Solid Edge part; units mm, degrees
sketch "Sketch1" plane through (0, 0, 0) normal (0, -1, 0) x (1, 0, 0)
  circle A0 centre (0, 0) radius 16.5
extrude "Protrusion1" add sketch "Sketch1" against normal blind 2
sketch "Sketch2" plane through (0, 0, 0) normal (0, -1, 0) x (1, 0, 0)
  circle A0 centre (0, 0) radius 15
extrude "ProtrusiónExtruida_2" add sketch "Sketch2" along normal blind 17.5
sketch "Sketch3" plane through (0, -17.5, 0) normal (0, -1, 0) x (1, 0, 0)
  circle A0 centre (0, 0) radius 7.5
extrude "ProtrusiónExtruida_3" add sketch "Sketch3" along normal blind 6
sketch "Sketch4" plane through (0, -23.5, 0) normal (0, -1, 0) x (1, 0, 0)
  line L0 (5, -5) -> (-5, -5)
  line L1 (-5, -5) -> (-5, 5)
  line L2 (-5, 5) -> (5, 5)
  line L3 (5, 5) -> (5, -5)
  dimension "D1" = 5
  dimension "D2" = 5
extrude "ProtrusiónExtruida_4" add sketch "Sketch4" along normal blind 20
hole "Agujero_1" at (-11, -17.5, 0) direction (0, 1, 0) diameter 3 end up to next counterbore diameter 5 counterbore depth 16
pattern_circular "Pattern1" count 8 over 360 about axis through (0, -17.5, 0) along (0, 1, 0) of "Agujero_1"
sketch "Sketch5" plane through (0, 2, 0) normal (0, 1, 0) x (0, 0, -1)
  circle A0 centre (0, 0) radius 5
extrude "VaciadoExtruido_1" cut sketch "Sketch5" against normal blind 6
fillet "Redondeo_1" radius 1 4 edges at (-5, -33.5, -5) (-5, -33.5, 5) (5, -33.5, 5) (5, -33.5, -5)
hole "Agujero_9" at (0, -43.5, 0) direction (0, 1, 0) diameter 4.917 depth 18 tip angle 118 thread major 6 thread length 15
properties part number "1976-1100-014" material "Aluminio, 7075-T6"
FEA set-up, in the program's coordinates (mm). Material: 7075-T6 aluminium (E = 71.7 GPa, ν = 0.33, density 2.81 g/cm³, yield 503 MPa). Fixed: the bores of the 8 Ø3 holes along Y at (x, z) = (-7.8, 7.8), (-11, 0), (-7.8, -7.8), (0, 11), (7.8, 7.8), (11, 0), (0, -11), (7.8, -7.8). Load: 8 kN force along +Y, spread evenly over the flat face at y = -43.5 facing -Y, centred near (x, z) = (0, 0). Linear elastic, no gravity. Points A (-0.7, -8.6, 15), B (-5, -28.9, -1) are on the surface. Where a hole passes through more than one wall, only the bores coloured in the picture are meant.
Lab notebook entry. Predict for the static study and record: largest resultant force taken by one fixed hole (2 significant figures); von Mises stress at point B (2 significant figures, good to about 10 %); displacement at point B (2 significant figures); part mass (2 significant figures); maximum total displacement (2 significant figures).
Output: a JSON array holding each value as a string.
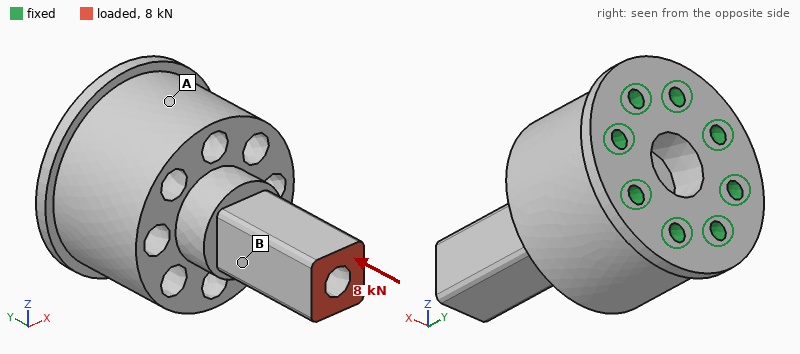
["1.1 kN", "98 MPa", "20 µm", "38 g", "40 µm"]
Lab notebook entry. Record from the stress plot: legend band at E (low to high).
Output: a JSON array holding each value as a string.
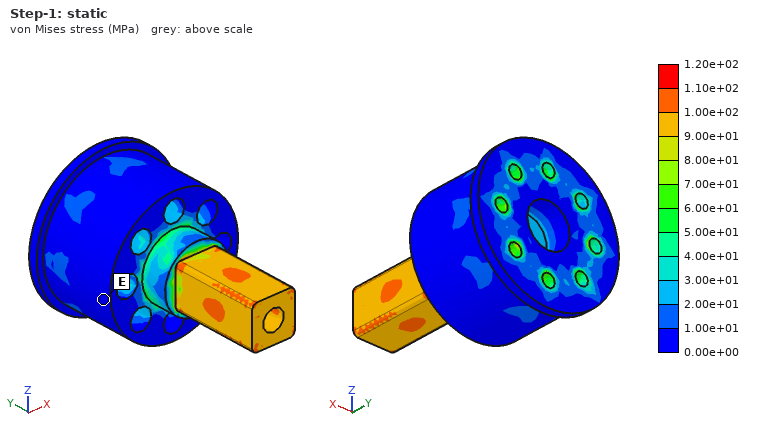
["0.00e+00 to 1.00e+01 MPa"]
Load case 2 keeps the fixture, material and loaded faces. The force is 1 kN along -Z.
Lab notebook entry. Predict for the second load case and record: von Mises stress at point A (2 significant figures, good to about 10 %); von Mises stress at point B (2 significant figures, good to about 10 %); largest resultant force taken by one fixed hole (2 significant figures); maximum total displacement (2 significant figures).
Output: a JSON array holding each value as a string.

["12 MPa", "44 MPa", "940 N", "0.12 mm"]
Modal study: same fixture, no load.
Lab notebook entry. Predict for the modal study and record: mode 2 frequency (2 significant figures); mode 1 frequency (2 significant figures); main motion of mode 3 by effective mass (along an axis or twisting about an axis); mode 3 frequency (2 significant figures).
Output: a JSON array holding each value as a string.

["11 kHz", "11 kHz", "along X", "24 kHz"]
